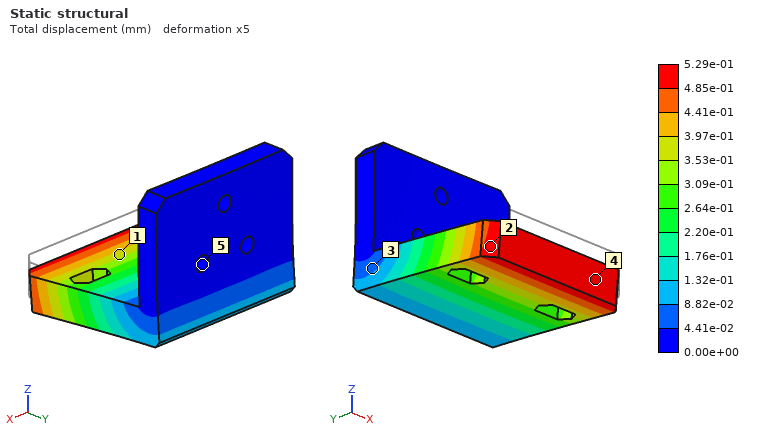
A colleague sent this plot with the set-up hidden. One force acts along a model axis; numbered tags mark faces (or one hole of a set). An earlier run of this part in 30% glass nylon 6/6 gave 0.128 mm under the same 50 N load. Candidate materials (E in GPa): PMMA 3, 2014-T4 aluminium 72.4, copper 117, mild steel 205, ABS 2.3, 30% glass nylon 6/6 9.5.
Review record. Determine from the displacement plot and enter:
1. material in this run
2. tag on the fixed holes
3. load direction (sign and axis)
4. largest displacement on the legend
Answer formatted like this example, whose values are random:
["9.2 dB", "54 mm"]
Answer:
["ABS", "5", "-Z", "5.29e-01 mm"]
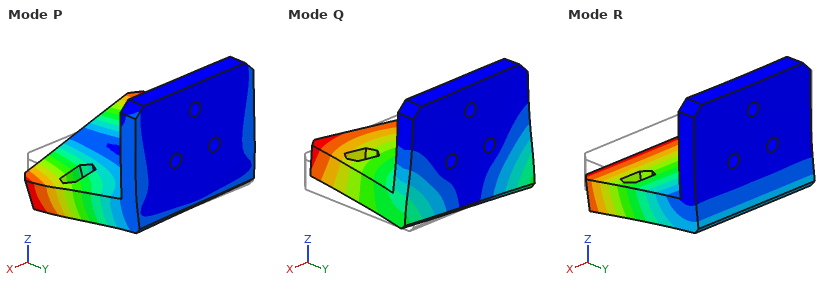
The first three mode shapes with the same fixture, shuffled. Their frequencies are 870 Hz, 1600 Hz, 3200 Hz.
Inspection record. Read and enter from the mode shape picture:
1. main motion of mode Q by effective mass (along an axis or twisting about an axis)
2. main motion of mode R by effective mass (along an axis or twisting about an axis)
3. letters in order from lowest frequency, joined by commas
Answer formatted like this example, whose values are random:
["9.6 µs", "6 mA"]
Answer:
["along X", "along Z", "R, Q, P"]
